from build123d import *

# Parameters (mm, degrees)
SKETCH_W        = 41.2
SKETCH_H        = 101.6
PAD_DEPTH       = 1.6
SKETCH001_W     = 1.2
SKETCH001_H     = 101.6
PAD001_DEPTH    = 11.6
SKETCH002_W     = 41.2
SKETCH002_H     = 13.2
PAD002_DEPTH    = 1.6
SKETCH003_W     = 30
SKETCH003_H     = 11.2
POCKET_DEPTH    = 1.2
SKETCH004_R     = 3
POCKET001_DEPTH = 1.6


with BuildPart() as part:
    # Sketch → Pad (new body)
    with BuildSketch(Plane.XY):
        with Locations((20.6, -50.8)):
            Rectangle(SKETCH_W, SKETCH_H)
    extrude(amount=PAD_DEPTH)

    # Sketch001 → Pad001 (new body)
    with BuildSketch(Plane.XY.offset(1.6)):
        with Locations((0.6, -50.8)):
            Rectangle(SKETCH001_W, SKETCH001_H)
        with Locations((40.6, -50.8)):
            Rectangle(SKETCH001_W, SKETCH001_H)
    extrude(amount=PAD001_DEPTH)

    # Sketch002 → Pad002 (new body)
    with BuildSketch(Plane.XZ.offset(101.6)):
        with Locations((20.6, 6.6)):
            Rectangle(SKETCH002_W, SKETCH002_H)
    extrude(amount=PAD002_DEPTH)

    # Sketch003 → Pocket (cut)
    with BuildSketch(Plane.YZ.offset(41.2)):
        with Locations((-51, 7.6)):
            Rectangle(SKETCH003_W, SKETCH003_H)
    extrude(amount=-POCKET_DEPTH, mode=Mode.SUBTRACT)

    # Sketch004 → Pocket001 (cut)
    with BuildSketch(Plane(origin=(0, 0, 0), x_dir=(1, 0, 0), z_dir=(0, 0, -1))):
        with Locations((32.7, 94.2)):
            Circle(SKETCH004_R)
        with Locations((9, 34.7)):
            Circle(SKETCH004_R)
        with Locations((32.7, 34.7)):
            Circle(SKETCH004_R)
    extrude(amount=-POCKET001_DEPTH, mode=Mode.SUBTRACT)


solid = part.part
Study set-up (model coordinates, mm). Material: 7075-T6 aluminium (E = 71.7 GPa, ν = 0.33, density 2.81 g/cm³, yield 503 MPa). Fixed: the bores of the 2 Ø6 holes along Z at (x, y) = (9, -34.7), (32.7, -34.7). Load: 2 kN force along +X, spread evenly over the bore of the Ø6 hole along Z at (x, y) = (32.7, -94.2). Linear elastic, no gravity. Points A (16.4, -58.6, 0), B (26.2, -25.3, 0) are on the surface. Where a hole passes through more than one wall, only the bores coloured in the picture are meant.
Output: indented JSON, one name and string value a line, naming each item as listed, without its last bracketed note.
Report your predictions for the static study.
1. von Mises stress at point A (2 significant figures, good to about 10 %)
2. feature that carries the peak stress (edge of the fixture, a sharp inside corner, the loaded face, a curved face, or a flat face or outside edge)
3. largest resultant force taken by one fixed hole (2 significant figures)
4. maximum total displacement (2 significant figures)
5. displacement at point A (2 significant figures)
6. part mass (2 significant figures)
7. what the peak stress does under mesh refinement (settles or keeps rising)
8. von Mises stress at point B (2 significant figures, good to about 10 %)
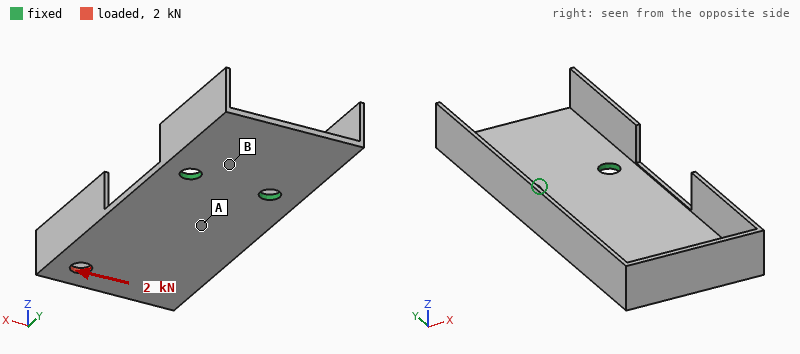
{
  "von Mises stress at point A": "87 MPa",
  "feature that carries the peak stress": "edge of the fixture",
  "largest resultant force taken by one fixed hole": "4.5 kN",
  "maximum total displacement": "0.50 mm",
  "displacement at point A": "0.092 mm",
  "part mass": "28 g",
  "what the peak stress does under mesh refinement": "keeps rising",
  "von Mises stress at point B": "28 MPa"
}
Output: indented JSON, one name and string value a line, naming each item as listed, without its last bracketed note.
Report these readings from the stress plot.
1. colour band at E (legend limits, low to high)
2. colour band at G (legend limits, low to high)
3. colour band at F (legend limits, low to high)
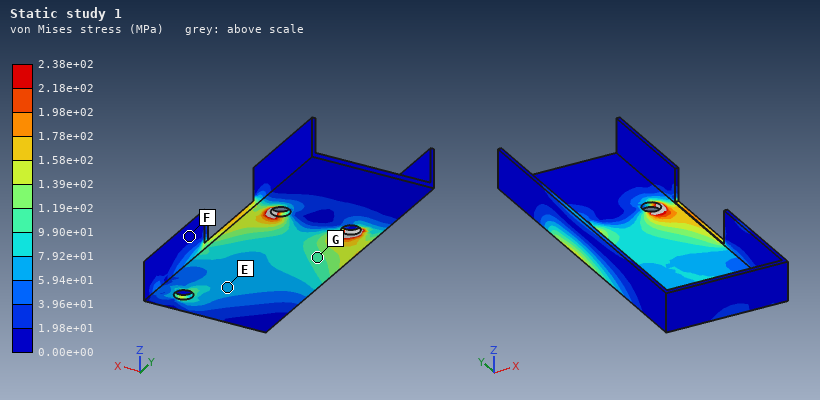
{
  "colour band at E": "5.94e+01 to 7.92e+01 MPa",
  "colour band at G": "9.90e+01 to 1.19e+02 MPa",
  "colour band at F": "0.00e+00 to 1.98e+01 MPa"
}
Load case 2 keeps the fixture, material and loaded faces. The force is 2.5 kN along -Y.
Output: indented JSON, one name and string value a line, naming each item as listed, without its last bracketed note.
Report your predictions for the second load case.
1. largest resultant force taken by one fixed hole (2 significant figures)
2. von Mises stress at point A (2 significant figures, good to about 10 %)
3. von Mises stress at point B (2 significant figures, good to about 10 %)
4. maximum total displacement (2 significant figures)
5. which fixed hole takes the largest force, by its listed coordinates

{
  "largest resultant force taken by one fixed hole": "2.4 kN",
  "von Mises stress at point A": "23 MPa",
  "von Mises stress at point B": "14 MPa",
  "maximum total displacement": "0.13 mm",
  "which fixed hole takes the largest force, by its listed coordinates": "(32.7, -34.7)"
}
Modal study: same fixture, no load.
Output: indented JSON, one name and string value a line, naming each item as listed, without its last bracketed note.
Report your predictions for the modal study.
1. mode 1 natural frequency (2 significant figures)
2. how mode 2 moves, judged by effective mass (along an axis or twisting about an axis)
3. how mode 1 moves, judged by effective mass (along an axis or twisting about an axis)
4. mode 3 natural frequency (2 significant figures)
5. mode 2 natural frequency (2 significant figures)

{
  "mode 1 natural frequency": "410 Hz",
  "how mode 2 moves, judged by effective mass": "twisting about Y",
  "how mode 1 moves, judged by effective mass": "along Z",
  "mode 3 natural frequency": "1800 Hz",
  "mode 2 natural frequency": "840 Hz"
}
